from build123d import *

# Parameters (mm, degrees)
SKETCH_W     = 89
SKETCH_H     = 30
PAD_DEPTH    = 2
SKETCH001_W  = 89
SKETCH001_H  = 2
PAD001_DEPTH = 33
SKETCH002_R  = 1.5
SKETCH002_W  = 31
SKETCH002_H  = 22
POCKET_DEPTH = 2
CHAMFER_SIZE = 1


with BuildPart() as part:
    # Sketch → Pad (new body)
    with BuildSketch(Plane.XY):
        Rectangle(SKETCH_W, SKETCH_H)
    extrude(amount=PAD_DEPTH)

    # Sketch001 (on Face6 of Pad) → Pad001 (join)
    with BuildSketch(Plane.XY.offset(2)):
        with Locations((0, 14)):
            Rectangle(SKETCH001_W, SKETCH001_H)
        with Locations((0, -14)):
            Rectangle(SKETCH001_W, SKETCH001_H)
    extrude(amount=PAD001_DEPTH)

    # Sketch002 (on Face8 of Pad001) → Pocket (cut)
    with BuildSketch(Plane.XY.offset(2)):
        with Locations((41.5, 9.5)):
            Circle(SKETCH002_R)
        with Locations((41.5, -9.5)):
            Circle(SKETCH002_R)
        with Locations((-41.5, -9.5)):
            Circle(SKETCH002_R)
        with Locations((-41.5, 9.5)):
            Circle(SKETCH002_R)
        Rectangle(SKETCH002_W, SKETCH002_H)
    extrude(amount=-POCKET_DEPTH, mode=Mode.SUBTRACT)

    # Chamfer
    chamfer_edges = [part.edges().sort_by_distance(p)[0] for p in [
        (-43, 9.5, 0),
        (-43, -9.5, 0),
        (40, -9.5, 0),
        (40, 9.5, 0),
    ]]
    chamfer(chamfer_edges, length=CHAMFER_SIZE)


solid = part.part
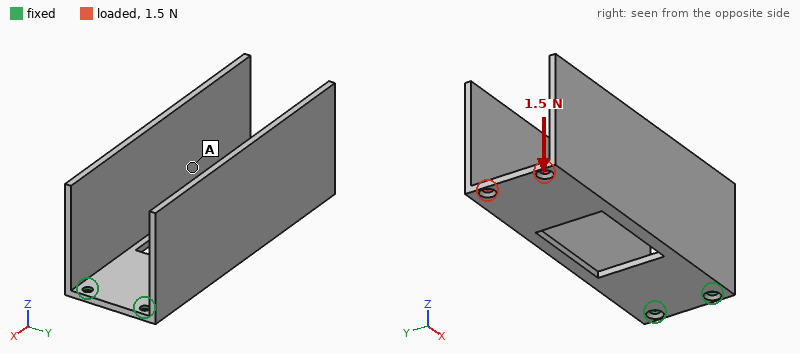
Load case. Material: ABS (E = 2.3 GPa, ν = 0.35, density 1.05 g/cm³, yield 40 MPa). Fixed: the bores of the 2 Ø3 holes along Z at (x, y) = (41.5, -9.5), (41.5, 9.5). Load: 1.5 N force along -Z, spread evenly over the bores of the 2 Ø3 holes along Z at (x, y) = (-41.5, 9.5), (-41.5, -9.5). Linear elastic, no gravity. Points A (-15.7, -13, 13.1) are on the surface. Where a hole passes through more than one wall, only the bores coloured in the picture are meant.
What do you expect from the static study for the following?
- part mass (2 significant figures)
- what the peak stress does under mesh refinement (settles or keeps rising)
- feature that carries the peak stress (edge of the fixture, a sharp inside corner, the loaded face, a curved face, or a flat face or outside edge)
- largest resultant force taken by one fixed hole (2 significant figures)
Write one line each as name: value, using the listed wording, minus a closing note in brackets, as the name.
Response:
part mass: 16 g
what the peak stress does under mesh refinement: keeps rising
feature that carries the peak stress: edge of the fixture
largest resultant force taken by one fixed hole: 1.1 N
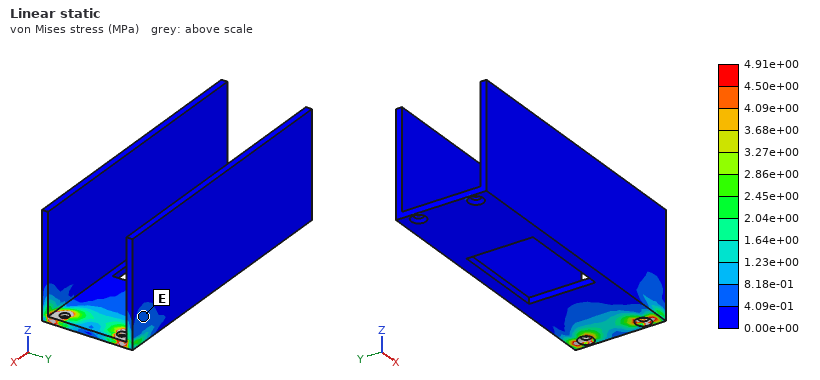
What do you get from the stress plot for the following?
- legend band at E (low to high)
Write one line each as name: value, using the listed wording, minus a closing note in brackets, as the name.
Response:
legend band at E: 4.09e-01 to 8.18e-01 MPa
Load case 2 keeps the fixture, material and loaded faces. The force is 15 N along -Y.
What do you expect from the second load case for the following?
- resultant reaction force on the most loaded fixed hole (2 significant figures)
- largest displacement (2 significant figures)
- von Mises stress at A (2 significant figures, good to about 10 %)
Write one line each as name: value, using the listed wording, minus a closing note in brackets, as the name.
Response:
resultant reaction force on the most loaded fixed hole: 60 N
largest displacement: 0.99 mm
von Mises stress at A: 1.8 MPa
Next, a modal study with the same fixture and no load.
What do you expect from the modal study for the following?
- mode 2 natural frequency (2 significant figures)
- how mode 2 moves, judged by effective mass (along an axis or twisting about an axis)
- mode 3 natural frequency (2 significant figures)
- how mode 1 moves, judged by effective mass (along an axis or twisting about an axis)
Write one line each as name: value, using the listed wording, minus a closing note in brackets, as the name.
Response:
mode 2 natural frequency: 120 Hz
how mode 2 moves, judged by effective mass: along Y
mode 3 natural frequency: 230 Hz
how mode 1 moves, judged by effective mass: along Z
